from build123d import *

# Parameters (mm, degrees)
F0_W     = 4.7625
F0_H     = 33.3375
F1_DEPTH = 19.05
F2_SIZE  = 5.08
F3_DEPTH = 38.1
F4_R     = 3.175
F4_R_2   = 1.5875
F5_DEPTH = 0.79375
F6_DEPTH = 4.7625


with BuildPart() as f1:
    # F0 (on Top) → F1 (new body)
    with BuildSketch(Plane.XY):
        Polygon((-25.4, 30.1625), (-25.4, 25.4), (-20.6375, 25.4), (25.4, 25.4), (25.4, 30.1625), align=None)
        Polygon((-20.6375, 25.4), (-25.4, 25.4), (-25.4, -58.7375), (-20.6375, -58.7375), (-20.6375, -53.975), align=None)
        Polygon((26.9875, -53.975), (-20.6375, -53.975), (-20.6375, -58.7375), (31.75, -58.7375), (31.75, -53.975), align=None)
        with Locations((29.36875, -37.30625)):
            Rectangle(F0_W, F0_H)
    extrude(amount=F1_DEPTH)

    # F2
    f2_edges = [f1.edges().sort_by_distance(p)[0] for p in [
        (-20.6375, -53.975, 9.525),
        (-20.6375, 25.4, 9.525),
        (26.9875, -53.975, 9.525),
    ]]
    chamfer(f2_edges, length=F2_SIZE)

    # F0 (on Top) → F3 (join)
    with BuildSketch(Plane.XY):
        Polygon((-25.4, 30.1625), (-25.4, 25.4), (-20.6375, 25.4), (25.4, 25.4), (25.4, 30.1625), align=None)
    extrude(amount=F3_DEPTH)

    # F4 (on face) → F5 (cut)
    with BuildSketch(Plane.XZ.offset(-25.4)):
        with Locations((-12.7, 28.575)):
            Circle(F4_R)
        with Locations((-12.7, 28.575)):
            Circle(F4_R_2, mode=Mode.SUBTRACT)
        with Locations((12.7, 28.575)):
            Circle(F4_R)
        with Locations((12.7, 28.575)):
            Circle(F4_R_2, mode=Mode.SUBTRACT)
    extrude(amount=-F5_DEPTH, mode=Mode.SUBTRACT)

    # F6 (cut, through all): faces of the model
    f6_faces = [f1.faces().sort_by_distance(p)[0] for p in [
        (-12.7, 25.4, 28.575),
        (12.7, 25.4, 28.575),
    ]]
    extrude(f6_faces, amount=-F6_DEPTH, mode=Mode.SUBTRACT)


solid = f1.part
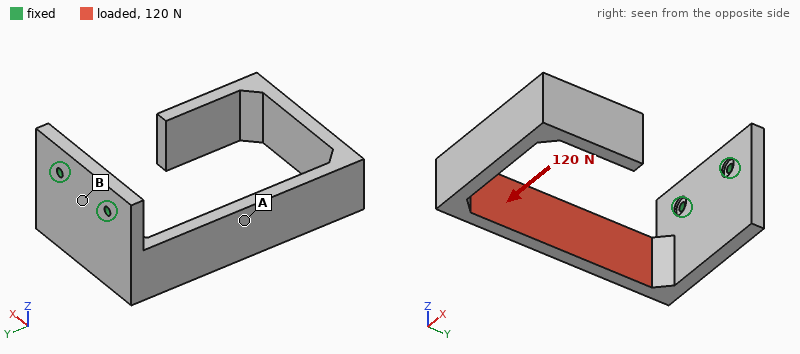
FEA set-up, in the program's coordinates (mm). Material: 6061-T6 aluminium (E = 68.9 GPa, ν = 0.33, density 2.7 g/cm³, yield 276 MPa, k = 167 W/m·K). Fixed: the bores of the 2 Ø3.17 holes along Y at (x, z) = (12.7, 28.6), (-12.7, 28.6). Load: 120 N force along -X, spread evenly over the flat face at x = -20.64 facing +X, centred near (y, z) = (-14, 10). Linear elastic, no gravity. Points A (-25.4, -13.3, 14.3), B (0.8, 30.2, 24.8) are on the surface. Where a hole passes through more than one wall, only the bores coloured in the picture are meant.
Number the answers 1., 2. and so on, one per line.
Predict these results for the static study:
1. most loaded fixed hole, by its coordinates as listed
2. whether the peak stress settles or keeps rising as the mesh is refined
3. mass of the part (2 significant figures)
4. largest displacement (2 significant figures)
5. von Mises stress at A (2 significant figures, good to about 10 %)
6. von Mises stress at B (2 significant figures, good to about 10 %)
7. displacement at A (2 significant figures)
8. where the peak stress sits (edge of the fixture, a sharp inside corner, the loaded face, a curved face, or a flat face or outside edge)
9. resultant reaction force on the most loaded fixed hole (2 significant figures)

1. (12.7, 28.6)
2. keeps rising
3. 68 g
4. 1.1 mm
5. 16 MPa
6. 6.1 MPa
7. 0.32 mm
8. edge of the fixture
9. 190 N
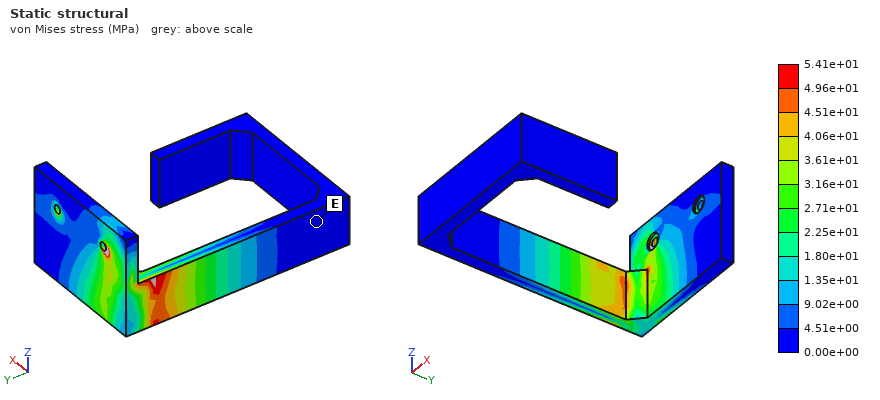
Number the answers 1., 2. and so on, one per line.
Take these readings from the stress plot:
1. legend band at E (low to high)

1. 0.00e+00 to 4.51e+00 MPa
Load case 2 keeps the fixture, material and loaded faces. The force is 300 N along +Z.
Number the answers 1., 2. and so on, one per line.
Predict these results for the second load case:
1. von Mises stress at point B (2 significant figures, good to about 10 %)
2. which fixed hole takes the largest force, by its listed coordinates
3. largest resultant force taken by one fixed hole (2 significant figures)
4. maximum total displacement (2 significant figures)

1. 46 MPa
2. (-12.7, 28.6)
3. 380 N
4. 1.3 mm
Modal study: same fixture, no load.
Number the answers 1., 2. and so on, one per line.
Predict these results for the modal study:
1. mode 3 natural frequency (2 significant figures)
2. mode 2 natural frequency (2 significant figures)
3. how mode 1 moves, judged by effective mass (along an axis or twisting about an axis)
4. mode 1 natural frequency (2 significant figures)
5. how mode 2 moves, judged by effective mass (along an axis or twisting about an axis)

1. 510 Hz
2. 270 Hz
3. along X
4. 200 Hz
5. along Z
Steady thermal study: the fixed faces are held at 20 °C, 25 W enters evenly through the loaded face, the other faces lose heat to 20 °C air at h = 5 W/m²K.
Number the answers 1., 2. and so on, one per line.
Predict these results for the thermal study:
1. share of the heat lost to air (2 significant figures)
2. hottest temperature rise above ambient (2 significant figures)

1. 9.9 %
2. 76 K
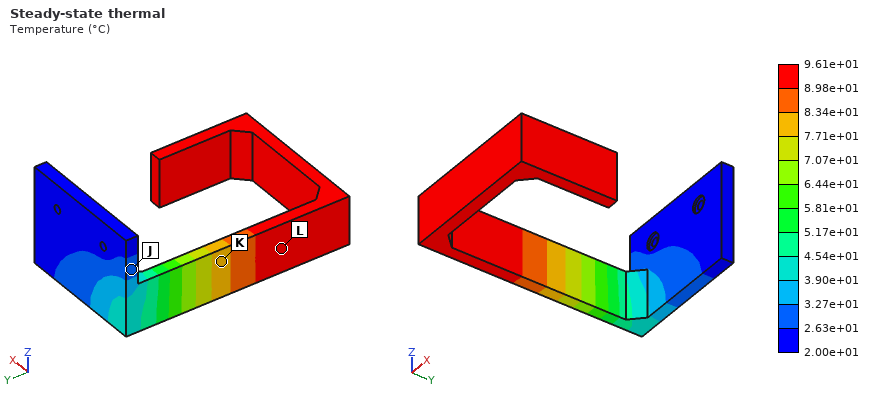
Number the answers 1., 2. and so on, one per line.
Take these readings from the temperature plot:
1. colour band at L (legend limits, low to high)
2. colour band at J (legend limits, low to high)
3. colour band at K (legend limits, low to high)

1. 8.98e+01 to 9.61e+01 °C
2. 2.63e+01 to 3.27e+01 °C
3. 7.71e+01 to 8.34e+01 °C
